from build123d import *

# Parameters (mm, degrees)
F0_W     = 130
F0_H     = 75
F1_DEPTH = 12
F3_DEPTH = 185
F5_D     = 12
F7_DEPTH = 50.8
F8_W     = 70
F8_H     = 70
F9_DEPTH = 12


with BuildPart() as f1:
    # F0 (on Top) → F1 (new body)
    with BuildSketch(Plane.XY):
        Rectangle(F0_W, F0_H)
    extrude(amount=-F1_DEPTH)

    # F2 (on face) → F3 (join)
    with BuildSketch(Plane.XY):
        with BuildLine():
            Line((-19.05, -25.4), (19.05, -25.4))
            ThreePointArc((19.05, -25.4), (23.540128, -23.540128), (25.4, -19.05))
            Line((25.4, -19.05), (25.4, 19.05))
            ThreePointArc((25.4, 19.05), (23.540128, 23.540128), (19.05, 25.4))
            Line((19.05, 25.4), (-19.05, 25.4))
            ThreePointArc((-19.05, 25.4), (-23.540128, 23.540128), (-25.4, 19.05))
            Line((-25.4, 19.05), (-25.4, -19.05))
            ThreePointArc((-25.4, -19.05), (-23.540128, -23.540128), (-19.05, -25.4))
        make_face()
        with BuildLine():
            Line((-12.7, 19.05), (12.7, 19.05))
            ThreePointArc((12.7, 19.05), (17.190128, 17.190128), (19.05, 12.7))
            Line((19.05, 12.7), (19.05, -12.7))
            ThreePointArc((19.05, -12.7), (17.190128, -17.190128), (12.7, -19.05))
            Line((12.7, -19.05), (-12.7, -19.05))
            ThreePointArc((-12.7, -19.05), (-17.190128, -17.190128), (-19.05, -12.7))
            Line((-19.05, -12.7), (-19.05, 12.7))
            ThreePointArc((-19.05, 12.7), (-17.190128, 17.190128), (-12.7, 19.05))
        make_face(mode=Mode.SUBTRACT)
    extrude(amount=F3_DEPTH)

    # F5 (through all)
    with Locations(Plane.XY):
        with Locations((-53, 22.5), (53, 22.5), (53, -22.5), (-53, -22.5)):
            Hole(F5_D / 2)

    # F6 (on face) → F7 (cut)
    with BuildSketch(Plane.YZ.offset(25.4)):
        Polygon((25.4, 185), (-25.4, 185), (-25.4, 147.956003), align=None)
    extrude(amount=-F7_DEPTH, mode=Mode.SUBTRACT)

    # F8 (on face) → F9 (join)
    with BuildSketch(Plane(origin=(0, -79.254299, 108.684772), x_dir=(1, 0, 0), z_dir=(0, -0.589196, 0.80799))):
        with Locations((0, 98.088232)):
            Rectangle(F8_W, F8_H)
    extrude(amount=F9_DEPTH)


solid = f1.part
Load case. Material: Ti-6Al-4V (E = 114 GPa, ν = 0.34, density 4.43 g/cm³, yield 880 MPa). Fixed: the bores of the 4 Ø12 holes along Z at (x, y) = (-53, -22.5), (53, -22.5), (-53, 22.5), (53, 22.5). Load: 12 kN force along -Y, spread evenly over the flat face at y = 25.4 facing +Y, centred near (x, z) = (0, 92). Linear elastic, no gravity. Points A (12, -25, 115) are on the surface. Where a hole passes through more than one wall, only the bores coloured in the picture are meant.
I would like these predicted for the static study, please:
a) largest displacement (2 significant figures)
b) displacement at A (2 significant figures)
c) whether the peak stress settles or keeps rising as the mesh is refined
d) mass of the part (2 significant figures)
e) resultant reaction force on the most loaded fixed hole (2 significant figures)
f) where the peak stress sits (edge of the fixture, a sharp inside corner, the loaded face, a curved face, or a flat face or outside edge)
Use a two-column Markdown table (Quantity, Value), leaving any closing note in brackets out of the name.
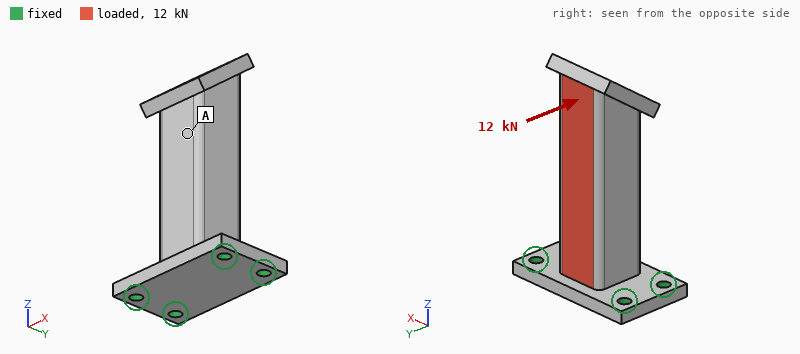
| Quantity | Value |
|---|---|
| largest displacement | 1.1 mm |
| displacement at A | 0.62 mm |
| whether the peak stress settles or keeps rising as the mesh is refined | keeps rising |
| mass of the part | 1.6 kg |
| resultant reaction force on the most loaded fixed hole | 13 kN |
| where the peak stress sits | edge of the fixture |
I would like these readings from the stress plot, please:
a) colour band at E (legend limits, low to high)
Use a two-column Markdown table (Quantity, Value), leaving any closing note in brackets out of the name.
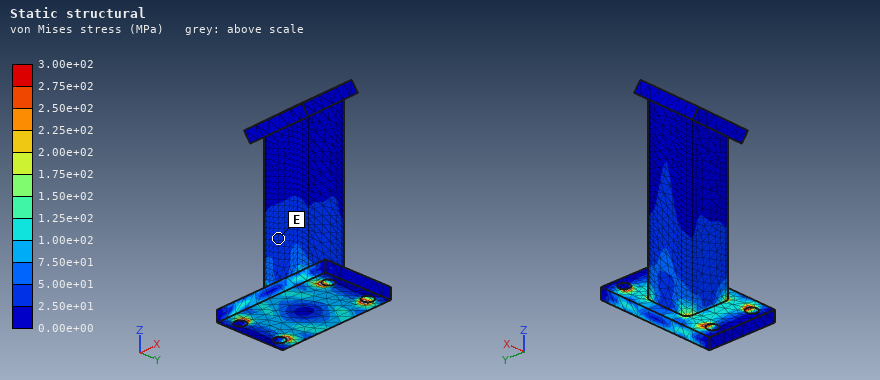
| Quantity | Value |
|---|---|
| colour band at E | 2.50e+01 to 5.00e+01 MPa |
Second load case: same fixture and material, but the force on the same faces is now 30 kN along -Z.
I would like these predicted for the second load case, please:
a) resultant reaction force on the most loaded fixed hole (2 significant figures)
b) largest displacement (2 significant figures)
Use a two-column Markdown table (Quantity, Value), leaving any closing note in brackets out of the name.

| Quantity | Value |
|---|---|
| resultant reaction force on the most loaded fixed hole | 15 kN |
| largest displacement | 0.74 mm |
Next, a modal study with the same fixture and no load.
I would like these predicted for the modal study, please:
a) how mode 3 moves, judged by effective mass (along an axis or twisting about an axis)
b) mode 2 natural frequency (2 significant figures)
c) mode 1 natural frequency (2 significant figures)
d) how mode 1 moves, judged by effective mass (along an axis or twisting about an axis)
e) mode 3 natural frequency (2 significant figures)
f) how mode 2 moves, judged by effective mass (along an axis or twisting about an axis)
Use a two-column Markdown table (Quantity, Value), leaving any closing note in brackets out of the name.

| Quantity | Value |
|---|---|
| how mode 3 moves, judged by effective mass | along Z |
| mode 2 natural frequency | 770 Hz |
| mode 1 natural frequency | 570 Hz |
| how mode 1 moves, judged by effective mass | along Y |
| mode 3 natural frequency | 2800 Hz |
| how mode 2 moves, judged by effective mass | along X |
